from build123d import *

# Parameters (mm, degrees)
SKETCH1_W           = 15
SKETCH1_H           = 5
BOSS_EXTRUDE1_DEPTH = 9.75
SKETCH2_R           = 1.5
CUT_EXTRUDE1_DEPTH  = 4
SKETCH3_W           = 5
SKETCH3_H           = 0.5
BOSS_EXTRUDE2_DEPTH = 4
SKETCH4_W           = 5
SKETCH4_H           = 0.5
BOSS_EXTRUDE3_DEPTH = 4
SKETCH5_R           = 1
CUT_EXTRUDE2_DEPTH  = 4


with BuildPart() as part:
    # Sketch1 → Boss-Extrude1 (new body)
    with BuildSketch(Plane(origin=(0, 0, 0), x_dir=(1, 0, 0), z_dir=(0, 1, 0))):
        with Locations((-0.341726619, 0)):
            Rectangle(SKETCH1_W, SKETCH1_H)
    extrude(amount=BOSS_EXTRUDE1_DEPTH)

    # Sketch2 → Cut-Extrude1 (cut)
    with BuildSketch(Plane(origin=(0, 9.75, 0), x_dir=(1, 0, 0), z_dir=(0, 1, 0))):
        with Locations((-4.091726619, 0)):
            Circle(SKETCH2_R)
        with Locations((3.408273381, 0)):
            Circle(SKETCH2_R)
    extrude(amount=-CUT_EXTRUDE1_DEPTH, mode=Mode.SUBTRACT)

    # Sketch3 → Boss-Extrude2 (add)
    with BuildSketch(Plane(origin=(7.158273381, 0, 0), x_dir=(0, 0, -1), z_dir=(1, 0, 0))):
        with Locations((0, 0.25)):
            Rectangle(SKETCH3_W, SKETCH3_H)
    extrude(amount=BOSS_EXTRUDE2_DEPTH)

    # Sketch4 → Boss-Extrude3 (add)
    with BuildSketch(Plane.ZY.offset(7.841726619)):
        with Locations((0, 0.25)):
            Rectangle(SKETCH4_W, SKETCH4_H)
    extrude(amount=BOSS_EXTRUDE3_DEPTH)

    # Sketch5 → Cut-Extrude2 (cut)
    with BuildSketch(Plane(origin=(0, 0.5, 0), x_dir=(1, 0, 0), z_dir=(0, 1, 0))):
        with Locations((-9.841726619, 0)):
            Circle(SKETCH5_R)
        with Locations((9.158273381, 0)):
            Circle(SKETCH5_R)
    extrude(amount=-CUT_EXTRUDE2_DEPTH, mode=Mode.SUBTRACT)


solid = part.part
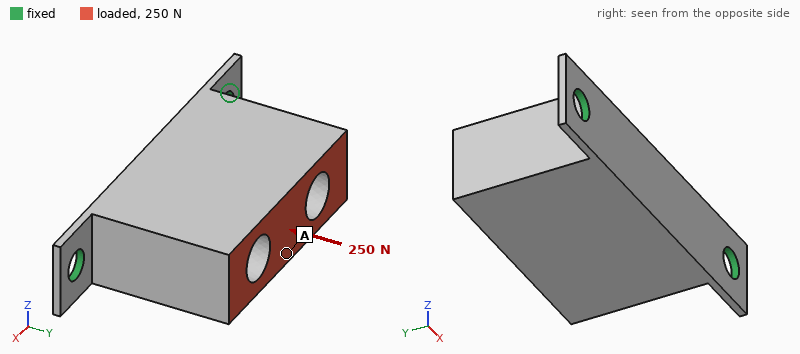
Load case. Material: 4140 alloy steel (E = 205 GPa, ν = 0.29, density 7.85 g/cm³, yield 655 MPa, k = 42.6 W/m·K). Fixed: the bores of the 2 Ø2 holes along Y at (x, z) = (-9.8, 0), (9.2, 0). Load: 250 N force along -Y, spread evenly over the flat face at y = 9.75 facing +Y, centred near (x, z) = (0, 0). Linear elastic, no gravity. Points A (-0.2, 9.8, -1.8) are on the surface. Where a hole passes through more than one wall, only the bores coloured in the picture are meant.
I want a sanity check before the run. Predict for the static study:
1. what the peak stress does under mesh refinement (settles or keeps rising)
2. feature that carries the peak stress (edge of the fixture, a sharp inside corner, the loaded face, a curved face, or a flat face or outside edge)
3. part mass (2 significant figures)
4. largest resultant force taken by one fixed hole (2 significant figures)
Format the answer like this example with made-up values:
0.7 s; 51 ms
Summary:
keeps rising; edge of the fixture; 5.4 g; 150 N
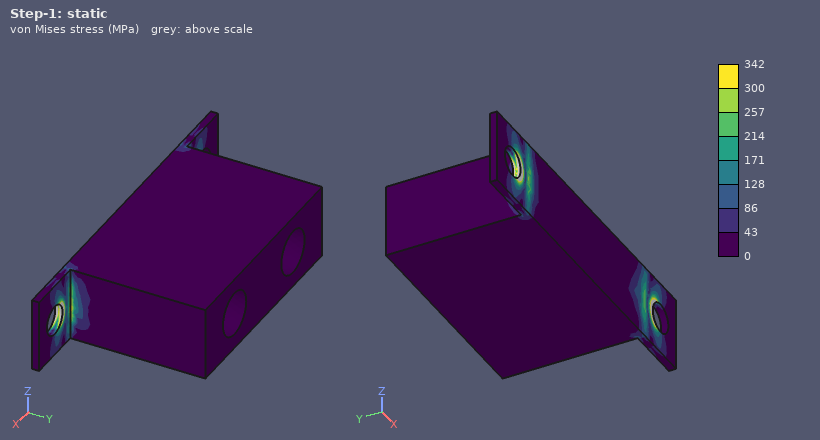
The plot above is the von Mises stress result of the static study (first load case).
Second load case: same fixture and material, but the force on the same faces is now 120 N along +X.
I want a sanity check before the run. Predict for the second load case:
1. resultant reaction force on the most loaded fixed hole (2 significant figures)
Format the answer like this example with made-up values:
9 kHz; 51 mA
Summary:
93 N
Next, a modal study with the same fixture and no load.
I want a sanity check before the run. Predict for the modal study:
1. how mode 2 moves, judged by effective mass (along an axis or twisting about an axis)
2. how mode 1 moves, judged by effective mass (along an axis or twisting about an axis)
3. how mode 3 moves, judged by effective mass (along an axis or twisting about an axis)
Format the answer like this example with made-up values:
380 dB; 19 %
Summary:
along Y; along Z; along X
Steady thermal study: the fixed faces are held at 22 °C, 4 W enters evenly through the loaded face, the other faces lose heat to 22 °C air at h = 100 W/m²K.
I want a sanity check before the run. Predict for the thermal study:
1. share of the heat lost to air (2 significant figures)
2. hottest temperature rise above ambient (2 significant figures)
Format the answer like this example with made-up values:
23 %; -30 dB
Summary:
41 %; 36 K
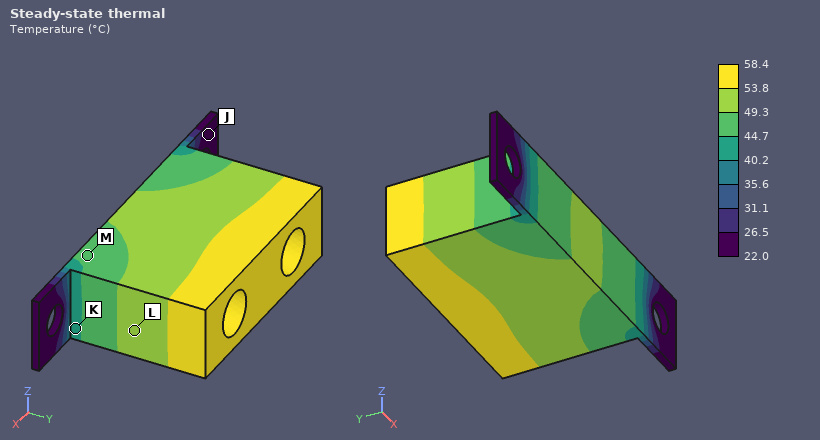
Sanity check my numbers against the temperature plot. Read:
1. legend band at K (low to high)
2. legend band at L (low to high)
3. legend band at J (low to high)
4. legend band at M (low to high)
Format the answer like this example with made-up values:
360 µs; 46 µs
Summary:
40.2 to 44.7 °C; 49.3 to 53.8 °C; 22.0 to 26.5 °C; 44.7 to 49.3 °C
